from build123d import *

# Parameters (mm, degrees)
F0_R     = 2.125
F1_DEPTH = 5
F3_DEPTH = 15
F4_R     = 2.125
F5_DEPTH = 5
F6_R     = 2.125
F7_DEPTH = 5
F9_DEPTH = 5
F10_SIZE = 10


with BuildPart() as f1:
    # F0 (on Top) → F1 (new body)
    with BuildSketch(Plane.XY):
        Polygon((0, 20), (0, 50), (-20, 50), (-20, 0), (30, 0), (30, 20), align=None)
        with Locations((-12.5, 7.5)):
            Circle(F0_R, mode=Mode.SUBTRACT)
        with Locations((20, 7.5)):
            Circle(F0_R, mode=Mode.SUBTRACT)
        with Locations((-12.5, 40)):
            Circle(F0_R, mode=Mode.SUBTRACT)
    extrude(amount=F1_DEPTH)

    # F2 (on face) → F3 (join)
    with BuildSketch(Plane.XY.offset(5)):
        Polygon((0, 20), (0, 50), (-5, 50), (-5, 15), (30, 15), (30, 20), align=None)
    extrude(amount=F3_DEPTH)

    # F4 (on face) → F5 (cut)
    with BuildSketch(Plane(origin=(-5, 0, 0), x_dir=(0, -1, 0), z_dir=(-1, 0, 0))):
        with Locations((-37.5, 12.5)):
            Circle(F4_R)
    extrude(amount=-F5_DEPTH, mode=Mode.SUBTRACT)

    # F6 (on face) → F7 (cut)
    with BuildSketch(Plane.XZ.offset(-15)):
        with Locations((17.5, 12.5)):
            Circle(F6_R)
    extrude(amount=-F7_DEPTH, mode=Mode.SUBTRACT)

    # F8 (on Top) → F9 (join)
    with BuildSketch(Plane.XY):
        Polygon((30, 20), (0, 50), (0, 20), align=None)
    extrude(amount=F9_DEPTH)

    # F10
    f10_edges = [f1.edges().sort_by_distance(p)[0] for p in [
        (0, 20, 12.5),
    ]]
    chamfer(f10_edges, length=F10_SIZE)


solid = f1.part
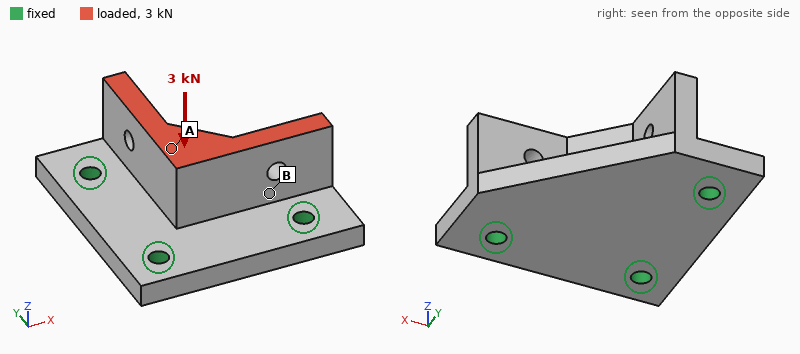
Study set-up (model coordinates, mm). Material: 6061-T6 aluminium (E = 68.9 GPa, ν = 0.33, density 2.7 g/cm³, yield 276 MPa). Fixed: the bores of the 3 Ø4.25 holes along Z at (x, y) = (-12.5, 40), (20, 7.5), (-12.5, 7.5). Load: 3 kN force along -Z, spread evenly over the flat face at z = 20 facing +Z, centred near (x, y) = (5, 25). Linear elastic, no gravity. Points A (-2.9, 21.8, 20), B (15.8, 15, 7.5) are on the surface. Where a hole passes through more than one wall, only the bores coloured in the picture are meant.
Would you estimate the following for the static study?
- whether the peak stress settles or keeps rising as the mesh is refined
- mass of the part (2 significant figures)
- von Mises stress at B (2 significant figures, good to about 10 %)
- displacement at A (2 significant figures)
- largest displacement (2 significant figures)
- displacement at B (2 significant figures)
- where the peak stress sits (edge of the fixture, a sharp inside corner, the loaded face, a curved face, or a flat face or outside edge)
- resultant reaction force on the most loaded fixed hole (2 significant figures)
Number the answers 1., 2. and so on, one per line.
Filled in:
1. keeps rising
2. 42 g
3. 44 MPa
4. 20 µm
5. 41 µm
6. 18 µm
7. edge of the fixture
8. 1.4 kN
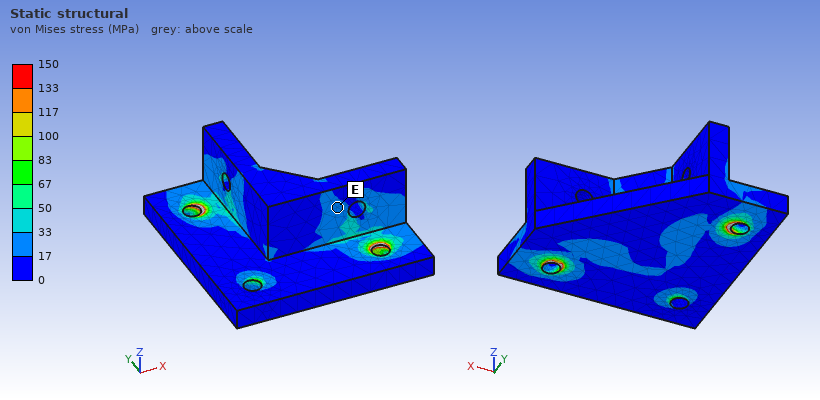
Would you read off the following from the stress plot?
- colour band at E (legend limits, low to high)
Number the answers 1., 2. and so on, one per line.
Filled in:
1. 17 to 33 MPa
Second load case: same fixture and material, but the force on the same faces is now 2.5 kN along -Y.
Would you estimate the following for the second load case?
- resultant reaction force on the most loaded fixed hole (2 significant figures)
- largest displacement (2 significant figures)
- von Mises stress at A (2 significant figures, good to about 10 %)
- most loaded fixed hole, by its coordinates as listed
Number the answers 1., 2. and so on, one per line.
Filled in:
1. 1.6 kN
2. 0.11 mm
3. 16 MPa
4. (-12.5, 40)
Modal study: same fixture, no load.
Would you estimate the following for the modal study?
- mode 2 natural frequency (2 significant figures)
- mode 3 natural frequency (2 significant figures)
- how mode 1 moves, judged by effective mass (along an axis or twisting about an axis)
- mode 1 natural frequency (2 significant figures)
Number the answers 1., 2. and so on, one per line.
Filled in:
1. 13 kHz
2. 14 kHz
3. along Z
4. 8300 Hz
